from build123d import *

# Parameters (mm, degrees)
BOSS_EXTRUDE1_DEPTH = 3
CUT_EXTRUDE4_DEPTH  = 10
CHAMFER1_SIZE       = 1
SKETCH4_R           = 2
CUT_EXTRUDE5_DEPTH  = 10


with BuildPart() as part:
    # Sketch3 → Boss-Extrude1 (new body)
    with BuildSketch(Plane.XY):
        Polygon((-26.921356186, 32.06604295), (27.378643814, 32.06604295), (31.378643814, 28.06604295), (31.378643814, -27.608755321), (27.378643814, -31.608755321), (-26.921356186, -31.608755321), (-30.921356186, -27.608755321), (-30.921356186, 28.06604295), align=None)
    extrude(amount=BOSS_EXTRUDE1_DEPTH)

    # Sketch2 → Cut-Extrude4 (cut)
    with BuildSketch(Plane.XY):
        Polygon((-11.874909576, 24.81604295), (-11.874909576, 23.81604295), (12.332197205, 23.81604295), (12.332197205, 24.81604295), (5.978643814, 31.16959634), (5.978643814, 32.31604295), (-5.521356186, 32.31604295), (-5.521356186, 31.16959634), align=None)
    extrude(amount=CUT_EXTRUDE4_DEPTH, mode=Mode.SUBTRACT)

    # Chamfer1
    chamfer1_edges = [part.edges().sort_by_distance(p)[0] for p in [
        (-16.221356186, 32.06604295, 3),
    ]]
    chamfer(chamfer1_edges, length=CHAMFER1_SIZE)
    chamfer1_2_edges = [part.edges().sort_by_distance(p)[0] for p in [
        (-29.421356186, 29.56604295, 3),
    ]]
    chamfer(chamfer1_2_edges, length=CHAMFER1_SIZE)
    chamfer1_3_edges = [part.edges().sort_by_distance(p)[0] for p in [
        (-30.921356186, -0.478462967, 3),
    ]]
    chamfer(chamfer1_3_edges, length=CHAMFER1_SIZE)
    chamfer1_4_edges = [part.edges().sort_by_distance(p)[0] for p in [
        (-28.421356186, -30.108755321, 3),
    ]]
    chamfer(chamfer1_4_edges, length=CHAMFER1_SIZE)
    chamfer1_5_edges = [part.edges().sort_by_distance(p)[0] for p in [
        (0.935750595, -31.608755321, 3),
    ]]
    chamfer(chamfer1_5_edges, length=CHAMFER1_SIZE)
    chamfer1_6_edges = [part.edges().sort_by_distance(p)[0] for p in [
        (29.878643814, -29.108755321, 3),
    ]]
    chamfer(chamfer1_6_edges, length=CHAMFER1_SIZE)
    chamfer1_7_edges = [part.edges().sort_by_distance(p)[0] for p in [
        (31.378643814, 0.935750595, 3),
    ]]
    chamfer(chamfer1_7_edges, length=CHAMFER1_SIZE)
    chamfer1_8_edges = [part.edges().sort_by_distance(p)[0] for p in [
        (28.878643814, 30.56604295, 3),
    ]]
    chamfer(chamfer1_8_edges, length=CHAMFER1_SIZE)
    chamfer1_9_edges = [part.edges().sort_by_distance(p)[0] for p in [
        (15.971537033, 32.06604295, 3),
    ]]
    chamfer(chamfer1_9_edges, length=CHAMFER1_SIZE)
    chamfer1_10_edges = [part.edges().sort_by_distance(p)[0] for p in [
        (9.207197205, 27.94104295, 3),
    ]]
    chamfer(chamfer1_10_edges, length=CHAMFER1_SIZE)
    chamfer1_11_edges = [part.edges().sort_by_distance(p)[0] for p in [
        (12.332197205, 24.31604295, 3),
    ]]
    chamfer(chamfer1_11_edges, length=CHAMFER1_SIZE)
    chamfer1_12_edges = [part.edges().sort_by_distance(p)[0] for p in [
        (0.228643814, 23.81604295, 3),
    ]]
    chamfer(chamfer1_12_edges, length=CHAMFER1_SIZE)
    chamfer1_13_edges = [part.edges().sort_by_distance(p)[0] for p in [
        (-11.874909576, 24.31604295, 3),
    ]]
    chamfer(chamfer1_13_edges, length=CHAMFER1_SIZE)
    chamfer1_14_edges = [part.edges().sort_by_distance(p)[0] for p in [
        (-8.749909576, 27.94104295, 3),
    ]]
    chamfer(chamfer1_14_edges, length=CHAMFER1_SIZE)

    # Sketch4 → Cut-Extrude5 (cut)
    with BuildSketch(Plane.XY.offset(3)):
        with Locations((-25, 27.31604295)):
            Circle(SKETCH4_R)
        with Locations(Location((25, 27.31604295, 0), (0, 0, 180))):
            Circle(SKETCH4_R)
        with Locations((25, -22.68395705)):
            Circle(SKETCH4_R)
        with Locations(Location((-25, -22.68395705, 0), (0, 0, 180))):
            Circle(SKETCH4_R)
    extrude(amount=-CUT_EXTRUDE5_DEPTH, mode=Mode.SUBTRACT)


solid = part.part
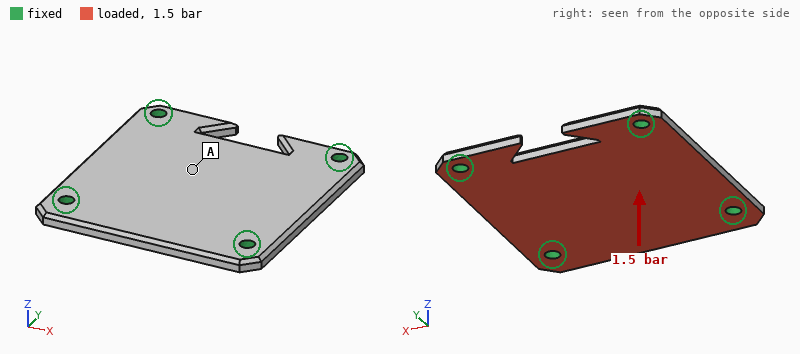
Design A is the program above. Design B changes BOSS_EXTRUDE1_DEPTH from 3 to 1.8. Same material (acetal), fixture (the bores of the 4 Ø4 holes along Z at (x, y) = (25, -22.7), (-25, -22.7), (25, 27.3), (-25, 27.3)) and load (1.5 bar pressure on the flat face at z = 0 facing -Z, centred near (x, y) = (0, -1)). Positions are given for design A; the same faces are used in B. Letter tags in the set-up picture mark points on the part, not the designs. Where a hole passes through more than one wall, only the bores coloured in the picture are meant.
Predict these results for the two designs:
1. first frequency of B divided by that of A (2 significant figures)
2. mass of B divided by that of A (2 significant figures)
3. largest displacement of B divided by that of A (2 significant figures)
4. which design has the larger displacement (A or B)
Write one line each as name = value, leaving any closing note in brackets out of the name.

first frequency of B divided by that of A = 0.62
mass of B divided by that of A = 0.60
largest displacement of B divided by that of A = 4.3
which design has the larger displacement = B
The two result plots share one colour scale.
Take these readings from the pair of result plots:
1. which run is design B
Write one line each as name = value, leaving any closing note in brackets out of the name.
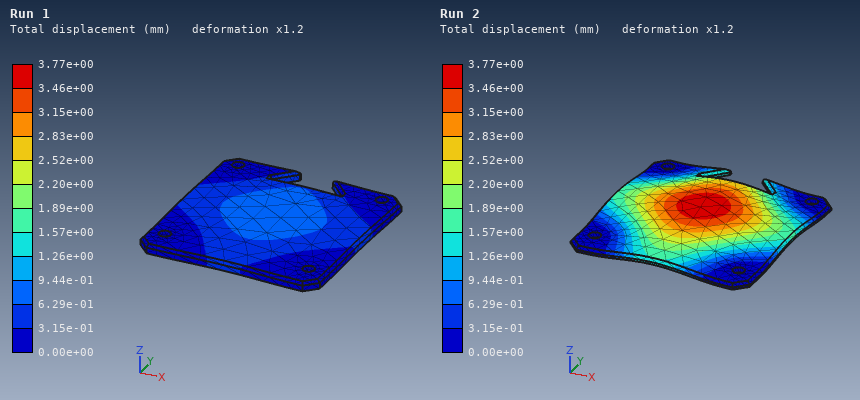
which run is design B = Run 2
